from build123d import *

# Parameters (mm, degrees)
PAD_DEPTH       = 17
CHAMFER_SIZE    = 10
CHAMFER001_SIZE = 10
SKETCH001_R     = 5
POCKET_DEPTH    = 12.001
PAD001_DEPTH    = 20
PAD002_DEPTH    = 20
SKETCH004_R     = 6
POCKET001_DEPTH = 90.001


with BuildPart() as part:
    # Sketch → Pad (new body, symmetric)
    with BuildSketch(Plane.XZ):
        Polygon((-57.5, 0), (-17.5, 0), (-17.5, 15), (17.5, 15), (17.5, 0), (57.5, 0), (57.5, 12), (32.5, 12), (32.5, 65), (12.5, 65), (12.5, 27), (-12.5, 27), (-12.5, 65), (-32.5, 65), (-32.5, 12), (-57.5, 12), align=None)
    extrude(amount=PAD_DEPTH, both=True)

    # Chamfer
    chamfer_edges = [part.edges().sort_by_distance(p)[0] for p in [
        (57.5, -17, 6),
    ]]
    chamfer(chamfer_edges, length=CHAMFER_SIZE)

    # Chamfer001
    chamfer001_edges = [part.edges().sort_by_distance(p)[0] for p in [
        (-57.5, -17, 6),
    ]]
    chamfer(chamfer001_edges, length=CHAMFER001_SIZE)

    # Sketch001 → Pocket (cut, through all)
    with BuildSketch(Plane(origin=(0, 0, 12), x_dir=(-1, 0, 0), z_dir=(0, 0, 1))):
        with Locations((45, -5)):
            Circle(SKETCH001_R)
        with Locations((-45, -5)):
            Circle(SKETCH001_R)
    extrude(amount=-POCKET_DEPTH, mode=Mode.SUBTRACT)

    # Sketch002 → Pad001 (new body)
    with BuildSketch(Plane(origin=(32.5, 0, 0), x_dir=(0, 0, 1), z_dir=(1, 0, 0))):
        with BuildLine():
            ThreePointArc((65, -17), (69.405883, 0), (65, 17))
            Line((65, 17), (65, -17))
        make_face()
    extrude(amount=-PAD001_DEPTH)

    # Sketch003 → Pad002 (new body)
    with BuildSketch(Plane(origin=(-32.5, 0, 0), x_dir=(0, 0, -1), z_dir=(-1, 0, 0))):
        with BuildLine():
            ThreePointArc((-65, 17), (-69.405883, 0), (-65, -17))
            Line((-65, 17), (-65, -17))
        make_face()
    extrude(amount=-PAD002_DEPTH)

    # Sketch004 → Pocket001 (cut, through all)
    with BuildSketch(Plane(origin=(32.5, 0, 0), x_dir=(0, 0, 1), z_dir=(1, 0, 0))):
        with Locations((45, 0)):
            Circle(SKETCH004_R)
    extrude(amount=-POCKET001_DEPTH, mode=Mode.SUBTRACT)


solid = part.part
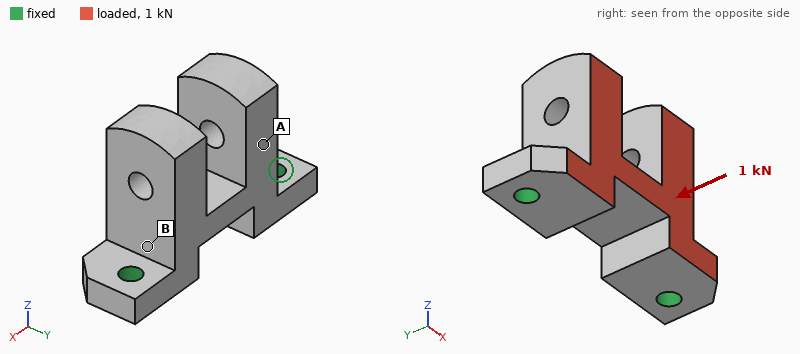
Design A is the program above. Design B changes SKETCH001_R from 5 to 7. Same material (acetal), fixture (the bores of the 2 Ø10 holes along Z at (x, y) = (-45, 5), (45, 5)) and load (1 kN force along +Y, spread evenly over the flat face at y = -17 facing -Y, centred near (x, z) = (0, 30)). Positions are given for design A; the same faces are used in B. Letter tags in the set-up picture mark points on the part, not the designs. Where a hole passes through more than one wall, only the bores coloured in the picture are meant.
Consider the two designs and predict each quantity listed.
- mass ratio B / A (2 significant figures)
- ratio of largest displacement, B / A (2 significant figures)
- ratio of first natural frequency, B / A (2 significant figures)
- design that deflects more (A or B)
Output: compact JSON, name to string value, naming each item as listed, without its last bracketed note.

{"mass ratio B / A": "0.98", "ratio of largest displacement, B / A": "0.76", "ratio of first natural frequency, B / A": "1.1", "design that deflects more": "A"}
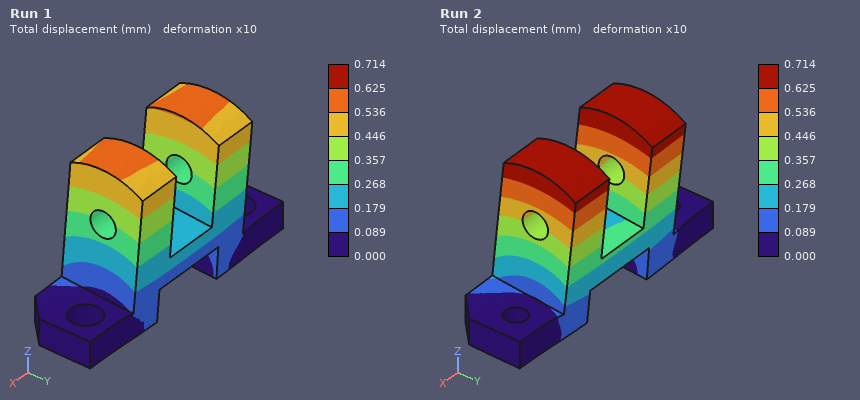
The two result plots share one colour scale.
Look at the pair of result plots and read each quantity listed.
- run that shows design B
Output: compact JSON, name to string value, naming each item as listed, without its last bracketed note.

{"run that shows design B": "Run 1"}
